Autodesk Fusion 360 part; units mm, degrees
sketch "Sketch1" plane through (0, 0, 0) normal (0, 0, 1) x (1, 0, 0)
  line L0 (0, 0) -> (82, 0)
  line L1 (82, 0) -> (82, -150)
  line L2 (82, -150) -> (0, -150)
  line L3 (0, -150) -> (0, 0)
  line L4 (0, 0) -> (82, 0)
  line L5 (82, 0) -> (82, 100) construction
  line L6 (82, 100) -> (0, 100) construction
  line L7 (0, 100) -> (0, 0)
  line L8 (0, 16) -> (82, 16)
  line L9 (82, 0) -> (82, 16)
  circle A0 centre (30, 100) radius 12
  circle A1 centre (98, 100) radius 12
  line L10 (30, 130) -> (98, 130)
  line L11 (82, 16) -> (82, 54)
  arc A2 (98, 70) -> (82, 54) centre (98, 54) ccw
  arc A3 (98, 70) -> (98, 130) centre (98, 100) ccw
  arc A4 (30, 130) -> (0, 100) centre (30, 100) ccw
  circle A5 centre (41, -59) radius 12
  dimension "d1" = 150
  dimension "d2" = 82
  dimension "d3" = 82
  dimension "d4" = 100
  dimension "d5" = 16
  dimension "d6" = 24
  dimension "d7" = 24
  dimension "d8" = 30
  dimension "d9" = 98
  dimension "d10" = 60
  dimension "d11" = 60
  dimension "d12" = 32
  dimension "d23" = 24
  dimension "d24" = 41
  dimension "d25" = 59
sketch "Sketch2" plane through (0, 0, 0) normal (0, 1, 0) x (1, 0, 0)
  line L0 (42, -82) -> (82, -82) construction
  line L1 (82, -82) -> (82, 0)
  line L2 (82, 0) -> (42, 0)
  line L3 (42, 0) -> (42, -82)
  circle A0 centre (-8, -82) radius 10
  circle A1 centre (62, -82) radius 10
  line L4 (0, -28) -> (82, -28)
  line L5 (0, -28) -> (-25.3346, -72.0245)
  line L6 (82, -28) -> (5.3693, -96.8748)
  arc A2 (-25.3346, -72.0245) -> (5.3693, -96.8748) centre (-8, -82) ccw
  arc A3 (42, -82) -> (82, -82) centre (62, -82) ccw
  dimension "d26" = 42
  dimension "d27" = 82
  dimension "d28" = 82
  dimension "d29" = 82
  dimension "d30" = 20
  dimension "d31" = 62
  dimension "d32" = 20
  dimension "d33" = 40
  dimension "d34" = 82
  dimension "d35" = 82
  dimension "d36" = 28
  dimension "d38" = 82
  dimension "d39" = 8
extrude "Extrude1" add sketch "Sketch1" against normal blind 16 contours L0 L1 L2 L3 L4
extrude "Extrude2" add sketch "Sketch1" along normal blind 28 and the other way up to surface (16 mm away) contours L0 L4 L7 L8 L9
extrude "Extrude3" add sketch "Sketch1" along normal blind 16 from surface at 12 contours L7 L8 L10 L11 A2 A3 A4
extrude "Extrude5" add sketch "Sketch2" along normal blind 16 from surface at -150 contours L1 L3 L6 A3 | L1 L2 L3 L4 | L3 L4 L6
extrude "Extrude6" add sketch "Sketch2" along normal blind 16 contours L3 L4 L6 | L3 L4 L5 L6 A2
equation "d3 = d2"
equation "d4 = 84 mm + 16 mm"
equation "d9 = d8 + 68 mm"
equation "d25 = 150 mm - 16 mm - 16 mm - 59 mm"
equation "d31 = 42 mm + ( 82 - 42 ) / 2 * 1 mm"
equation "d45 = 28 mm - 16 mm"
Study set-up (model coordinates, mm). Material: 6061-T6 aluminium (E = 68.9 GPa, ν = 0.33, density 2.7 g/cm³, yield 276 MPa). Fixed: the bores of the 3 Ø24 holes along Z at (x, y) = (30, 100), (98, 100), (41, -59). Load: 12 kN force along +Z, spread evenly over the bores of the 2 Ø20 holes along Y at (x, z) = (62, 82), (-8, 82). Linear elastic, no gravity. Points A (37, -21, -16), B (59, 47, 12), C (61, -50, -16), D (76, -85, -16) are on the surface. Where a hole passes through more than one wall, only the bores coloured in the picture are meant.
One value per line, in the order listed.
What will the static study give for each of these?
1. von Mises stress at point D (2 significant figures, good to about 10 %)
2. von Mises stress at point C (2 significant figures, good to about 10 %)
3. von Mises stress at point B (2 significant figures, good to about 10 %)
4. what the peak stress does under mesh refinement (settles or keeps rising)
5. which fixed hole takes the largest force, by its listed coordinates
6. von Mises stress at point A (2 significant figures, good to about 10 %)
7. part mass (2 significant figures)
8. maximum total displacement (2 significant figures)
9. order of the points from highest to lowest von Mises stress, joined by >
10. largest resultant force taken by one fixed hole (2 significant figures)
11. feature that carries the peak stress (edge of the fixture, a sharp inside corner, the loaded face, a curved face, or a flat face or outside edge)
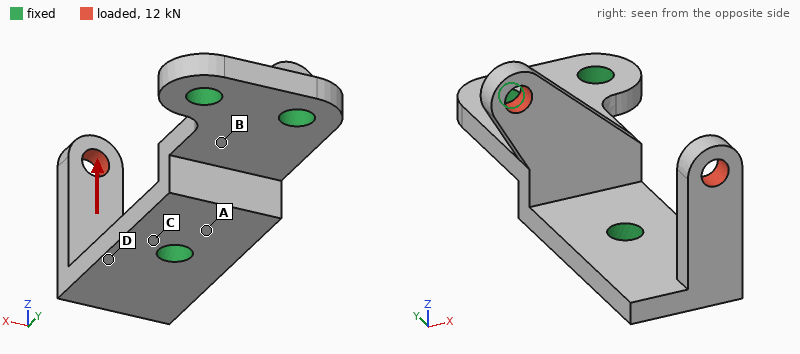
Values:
90 MPa
47 MPa
13 MPa
keeps rising
(41, -59)
30 MPa
1.5 kg
1.3 mm
D > C > A > B
11 kN
edge of the fixture
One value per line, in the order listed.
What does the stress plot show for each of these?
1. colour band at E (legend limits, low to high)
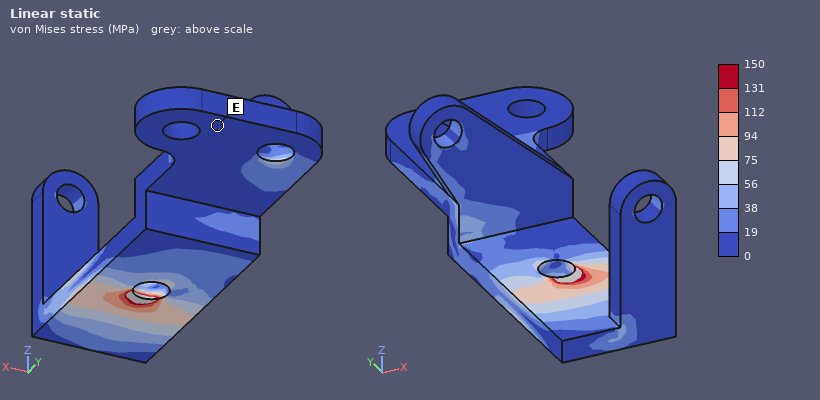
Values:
0 to 19 MPa
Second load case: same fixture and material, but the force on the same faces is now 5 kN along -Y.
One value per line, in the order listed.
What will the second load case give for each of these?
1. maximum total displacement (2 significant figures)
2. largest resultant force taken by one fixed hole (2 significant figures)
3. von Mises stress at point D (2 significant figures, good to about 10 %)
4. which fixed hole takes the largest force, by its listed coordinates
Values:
1.9 mm
4.8 kN
57 MPa
(30, 100)
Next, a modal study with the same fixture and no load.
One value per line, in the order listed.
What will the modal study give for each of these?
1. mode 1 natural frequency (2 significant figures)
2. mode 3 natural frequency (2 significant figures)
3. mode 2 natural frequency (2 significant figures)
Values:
700 Hz
1700 Hz
1000 Hz
